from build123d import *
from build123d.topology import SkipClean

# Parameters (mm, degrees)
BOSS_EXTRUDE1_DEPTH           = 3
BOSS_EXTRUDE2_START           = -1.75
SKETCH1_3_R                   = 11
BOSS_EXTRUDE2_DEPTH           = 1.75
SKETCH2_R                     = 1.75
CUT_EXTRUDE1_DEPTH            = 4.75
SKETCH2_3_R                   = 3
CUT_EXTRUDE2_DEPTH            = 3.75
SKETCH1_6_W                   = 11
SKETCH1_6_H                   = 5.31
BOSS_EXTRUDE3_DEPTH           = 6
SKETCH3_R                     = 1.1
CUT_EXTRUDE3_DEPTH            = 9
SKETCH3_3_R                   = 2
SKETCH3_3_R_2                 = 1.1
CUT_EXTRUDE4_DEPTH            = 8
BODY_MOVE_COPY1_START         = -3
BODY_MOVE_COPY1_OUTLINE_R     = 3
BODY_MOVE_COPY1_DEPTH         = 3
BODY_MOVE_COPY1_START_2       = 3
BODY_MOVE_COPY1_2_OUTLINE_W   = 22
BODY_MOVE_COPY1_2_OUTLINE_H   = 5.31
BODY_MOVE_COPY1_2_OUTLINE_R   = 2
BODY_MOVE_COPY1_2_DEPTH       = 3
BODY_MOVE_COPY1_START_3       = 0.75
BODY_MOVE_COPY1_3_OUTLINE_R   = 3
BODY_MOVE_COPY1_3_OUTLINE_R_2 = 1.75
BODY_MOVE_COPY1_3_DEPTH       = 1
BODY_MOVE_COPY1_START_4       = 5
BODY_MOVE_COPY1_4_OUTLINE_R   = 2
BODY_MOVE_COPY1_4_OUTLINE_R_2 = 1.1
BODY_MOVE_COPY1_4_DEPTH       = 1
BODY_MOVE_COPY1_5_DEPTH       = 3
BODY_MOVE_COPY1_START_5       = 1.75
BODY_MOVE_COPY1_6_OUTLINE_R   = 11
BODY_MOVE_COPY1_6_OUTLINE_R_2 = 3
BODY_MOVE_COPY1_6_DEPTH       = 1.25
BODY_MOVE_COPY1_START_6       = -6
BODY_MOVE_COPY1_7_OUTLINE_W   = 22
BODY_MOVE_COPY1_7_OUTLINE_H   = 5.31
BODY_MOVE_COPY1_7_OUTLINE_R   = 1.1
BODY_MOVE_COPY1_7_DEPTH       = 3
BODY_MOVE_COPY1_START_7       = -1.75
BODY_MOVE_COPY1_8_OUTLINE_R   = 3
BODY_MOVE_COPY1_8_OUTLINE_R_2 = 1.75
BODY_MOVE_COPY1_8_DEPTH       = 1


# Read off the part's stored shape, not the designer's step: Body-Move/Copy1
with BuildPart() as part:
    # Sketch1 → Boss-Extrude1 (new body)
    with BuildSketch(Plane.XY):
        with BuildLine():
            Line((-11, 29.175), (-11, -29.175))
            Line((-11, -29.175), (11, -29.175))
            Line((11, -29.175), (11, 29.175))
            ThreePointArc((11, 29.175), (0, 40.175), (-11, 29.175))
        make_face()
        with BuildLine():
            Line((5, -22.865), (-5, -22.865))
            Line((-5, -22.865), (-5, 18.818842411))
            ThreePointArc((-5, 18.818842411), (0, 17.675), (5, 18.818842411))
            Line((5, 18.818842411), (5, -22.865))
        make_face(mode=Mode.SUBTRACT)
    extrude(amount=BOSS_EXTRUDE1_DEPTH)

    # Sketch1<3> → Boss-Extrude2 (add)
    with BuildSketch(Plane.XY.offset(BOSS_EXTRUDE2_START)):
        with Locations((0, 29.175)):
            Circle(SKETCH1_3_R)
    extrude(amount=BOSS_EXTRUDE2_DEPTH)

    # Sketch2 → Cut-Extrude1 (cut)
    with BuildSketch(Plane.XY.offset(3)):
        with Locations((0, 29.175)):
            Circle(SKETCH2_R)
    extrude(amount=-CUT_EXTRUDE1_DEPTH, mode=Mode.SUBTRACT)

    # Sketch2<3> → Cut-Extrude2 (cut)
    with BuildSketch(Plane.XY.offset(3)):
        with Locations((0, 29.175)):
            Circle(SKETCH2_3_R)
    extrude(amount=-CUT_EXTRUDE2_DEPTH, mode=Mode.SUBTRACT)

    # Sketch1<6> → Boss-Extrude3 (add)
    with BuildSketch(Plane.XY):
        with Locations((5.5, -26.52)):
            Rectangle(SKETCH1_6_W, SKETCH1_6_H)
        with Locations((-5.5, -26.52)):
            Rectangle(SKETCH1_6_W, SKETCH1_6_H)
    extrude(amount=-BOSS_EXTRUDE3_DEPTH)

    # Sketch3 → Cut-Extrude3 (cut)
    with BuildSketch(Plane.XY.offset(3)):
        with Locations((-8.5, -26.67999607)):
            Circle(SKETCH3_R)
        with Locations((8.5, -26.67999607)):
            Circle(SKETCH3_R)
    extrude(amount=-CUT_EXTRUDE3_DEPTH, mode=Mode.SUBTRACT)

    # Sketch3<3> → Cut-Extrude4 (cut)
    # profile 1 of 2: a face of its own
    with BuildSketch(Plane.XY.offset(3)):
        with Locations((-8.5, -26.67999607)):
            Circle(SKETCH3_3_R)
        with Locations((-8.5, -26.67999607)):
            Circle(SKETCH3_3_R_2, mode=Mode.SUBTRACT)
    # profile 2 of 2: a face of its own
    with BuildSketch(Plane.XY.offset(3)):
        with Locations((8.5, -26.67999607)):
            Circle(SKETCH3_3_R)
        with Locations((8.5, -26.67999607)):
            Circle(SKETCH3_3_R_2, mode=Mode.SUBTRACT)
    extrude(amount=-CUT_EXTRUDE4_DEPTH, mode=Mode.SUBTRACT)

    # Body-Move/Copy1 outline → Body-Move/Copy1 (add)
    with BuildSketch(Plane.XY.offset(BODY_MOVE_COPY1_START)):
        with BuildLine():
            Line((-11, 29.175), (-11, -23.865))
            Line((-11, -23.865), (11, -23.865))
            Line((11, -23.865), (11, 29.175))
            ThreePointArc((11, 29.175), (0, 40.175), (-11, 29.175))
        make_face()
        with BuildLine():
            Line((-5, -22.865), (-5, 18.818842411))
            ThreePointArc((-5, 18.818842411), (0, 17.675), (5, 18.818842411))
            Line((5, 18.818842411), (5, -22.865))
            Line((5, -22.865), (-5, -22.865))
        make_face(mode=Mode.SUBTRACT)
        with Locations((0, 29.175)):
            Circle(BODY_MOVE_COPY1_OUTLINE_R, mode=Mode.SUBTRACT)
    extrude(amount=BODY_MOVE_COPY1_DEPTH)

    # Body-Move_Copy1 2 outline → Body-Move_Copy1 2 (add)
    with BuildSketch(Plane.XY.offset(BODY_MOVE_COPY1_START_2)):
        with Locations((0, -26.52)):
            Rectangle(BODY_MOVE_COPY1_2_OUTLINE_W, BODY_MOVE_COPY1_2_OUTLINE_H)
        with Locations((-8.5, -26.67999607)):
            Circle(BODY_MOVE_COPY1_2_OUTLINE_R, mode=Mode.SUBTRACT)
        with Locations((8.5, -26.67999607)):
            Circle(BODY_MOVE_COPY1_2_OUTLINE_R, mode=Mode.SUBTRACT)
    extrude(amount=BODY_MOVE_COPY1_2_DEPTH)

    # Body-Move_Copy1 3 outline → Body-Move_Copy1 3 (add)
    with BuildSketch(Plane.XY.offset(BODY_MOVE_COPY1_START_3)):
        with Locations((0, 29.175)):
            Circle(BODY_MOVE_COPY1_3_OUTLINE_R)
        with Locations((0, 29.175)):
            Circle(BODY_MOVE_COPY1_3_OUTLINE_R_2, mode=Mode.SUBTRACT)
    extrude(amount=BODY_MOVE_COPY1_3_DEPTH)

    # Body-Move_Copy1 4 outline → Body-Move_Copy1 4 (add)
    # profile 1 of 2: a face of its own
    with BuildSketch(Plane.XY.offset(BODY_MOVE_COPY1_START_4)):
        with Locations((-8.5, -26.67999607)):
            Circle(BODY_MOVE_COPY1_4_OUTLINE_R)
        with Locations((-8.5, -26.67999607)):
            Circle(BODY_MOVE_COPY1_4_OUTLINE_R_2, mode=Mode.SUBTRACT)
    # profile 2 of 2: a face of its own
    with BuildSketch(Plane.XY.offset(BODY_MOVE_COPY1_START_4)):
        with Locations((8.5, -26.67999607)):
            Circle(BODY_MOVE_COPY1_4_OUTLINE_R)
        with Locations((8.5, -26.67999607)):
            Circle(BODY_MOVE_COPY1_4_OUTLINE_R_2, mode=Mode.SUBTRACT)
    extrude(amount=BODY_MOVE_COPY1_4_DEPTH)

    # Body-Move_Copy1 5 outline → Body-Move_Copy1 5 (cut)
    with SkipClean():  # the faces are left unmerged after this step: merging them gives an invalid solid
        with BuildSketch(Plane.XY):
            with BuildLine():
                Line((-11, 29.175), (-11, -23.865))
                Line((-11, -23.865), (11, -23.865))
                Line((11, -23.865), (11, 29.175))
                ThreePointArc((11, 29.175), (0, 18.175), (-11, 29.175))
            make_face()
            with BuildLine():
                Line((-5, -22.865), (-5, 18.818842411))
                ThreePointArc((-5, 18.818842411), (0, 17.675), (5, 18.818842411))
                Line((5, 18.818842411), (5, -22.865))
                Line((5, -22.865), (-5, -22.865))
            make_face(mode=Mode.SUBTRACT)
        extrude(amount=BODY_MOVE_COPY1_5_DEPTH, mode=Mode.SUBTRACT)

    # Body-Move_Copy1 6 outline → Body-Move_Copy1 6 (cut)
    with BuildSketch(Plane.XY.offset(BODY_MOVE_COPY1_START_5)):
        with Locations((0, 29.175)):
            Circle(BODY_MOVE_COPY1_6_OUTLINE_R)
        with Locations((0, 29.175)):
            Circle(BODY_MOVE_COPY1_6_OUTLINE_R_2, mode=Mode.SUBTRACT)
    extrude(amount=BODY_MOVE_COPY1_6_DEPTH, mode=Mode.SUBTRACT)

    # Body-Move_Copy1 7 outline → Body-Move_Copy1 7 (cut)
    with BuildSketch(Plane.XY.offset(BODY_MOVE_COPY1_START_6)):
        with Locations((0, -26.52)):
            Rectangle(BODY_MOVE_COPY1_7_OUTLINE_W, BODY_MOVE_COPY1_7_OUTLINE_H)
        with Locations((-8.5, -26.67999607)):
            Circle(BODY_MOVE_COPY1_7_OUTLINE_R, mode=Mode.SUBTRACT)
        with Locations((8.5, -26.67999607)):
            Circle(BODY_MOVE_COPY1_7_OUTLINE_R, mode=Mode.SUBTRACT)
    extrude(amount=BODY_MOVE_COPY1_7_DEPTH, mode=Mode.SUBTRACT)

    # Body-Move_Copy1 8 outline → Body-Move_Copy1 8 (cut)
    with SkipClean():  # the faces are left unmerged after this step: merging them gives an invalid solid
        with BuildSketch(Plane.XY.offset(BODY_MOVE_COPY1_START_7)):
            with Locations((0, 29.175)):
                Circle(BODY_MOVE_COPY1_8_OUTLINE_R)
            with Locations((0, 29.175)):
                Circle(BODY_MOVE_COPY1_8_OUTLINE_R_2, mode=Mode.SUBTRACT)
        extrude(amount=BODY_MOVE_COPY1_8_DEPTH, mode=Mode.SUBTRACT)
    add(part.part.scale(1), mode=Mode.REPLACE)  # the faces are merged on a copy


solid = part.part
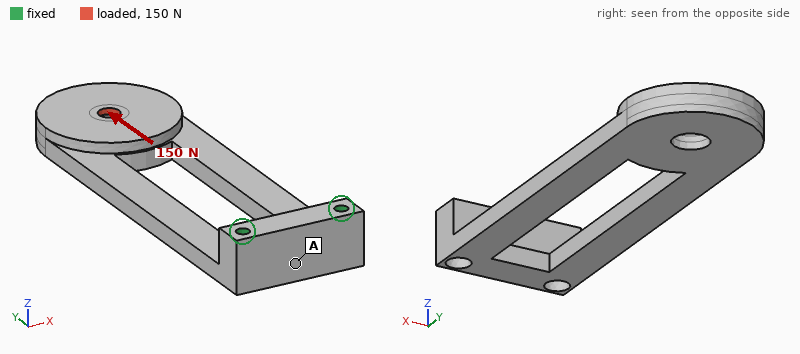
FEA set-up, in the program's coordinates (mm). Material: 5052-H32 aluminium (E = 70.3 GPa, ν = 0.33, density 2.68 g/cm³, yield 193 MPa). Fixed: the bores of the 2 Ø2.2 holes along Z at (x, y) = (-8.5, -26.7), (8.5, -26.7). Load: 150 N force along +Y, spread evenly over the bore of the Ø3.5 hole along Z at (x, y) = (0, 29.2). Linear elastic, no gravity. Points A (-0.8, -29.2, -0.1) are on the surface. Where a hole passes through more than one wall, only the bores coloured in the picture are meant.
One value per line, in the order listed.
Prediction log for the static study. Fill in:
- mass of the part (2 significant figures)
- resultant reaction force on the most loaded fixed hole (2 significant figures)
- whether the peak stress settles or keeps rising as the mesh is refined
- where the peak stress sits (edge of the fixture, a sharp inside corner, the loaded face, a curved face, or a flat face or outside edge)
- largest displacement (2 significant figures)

11 g
75 N
keeps rising
edge of the fixture
0.32 mm
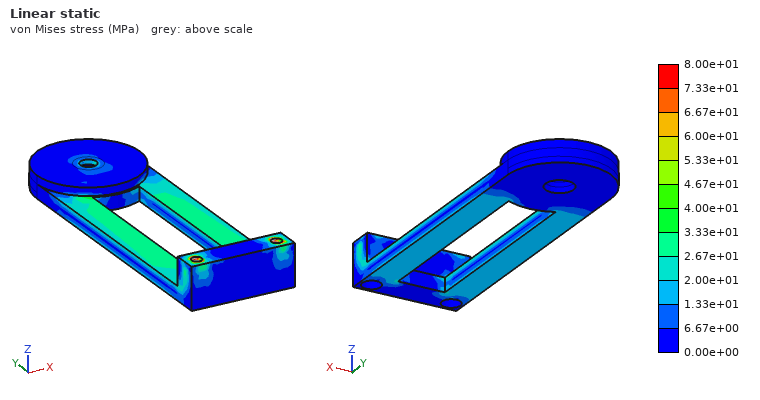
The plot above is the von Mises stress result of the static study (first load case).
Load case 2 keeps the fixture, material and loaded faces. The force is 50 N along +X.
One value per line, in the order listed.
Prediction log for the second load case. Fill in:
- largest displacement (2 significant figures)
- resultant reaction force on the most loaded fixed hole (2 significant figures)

0.18 mm
150 N
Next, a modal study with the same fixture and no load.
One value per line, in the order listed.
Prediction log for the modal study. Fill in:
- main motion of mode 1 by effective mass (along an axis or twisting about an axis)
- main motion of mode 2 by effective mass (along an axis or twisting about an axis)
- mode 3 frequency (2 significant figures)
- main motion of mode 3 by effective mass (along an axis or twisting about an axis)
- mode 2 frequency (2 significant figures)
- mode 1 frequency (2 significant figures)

along Z
along X
2200 Hz
twisting about Y
1200 Hz
350 Hz
